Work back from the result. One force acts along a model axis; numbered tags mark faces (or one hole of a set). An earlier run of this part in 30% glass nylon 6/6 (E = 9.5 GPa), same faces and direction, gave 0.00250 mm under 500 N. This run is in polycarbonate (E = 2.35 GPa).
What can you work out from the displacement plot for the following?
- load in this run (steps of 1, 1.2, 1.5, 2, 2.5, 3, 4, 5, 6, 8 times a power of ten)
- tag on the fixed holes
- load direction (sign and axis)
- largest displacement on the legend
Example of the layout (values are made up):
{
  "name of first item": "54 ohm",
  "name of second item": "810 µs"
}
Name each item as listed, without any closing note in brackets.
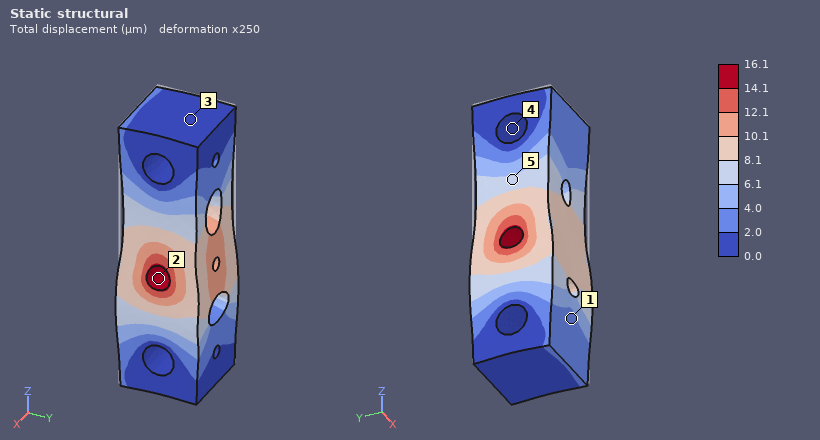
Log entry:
{
  "load in this run": "800 N",
  "tag on the fixed holes": "4",
  "load direction": "-Z",
  "largest displacement on the legend": "16.1 µm"
}
